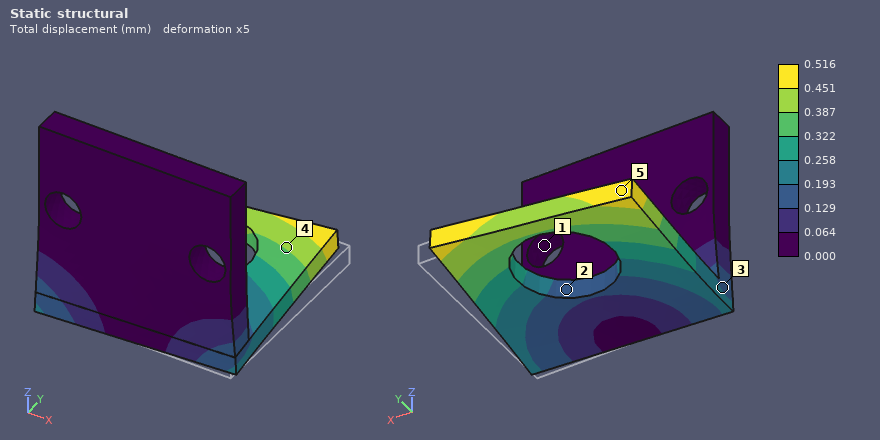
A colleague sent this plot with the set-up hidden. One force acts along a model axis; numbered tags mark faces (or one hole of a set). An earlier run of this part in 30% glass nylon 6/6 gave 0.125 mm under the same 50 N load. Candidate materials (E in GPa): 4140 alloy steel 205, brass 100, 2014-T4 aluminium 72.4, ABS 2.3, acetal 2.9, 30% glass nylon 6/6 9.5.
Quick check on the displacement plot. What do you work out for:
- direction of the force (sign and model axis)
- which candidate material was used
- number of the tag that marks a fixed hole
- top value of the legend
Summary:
-X
ABS
1
0.516 mm
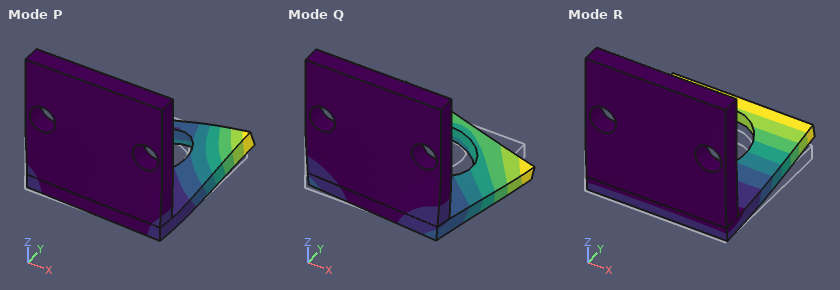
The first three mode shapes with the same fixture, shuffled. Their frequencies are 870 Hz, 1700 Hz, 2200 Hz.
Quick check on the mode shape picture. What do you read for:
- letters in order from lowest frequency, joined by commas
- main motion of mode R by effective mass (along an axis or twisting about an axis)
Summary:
R, Q, P
along Z
